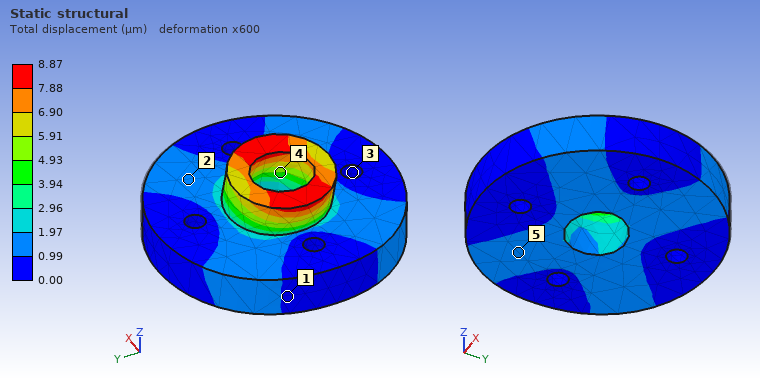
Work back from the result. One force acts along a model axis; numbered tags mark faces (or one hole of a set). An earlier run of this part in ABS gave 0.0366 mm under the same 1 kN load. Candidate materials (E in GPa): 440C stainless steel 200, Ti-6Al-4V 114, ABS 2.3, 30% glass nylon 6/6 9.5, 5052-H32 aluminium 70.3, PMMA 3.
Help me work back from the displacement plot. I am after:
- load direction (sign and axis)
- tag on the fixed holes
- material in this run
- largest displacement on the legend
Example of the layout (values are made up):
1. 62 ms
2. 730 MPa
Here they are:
1. -X
2. 3
3. 30% glass nylon 6/6
4. 8.87 µm
